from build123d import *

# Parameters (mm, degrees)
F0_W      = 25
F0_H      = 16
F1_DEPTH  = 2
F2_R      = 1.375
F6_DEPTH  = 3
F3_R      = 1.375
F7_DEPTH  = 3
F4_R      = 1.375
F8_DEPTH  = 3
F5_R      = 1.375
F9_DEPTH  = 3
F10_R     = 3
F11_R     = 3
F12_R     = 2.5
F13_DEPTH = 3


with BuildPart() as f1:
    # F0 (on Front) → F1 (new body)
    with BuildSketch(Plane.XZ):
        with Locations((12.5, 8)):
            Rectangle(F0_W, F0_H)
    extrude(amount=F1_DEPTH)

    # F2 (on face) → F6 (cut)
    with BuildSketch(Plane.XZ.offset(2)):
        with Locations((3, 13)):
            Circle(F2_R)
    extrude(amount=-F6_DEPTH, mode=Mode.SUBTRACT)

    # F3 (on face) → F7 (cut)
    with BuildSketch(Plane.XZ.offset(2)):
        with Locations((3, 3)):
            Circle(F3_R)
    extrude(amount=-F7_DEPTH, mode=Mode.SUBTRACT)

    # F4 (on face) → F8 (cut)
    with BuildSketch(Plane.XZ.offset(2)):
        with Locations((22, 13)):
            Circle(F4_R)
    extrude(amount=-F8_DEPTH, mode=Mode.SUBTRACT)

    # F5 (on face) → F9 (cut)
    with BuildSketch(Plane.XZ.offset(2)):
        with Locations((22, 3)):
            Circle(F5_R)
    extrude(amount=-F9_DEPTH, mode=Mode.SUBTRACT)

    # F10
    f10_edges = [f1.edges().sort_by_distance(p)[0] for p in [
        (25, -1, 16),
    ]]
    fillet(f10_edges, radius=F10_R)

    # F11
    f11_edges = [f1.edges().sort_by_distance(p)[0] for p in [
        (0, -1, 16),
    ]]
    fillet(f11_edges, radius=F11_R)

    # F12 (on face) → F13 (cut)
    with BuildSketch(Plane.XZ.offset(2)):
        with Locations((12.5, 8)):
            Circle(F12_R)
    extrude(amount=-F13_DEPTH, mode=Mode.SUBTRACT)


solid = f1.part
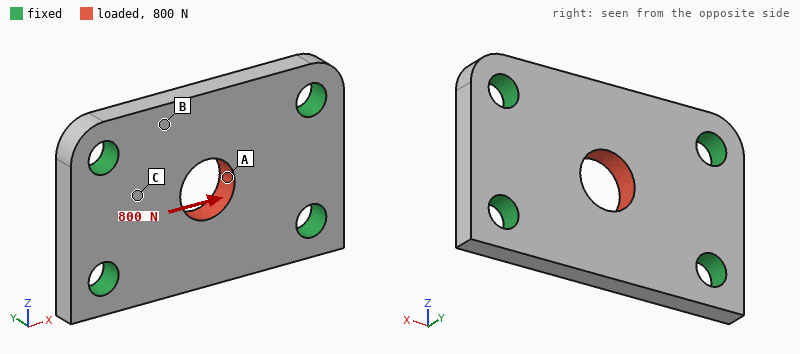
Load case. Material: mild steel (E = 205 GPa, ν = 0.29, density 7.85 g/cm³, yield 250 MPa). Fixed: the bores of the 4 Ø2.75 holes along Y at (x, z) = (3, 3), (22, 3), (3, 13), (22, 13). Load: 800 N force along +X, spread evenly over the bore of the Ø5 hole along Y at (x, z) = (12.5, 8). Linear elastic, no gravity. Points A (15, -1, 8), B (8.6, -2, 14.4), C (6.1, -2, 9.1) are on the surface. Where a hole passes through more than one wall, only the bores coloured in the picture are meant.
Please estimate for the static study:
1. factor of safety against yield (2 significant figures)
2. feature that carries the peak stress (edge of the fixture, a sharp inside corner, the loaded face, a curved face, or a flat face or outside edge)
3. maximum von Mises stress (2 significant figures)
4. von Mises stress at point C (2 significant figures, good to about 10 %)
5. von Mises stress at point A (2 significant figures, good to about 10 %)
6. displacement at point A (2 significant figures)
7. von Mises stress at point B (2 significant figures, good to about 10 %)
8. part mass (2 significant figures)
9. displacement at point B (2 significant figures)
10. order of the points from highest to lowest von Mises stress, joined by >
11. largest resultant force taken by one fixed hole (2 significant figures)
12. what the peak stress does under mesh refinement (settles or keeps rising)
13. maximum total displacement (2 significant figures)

5.7
the loaded face
44 MPa
15 MPa
23 MPa
0.77 µm
6.6 MPa
5.5 g
0.27 µm
A > C > B
210 N
settles
0.82 µm
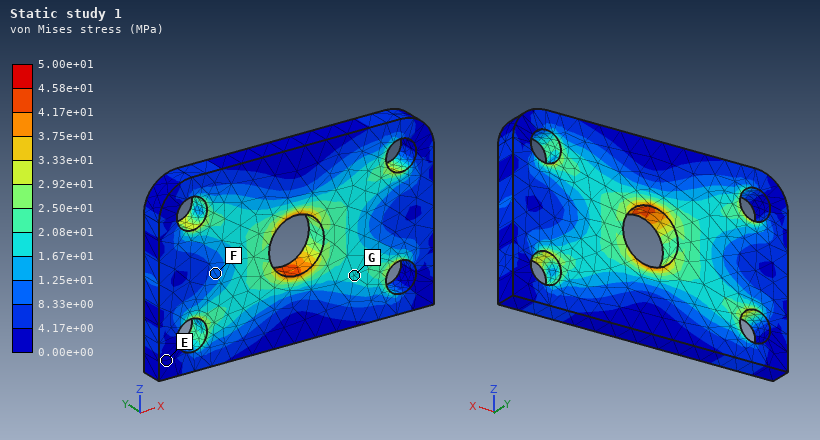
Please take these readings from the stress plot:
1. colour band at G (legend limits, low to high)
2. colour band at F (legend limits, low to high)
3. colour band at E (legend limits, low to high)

1.67e+01 to 2.08e+01 MPa
8.33e+00 to 1.25e+01 MPa
0.00e+00 to 4.17e+00 MPa
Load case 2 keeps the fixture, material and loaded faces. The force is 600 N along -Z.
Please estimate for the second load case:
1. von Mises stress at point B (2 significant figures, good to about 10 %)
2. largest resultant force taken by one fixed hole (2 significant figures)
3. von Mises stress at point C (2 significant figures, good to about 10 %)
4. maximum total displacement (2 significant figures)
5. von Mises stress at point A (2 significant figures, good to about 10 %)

11 MPa
180 N
20 MPa
1.3 µm
34 MPa
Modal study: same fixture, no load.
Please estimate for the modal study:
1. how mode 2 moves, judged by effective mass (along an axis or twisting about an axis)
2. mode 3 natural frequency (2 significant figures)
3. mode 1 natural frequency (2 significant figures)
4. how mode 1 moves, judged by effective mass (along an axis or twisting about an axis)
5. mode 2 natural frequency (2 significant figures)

twisting about X
60 kHz
32 kHz
along Y
38 kHz
